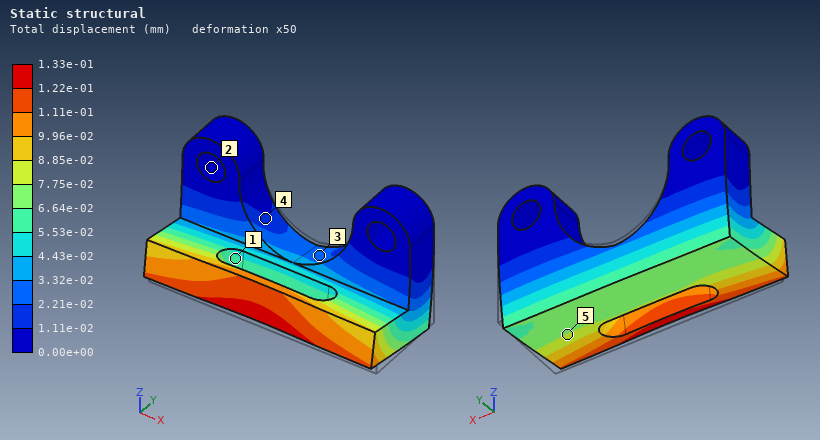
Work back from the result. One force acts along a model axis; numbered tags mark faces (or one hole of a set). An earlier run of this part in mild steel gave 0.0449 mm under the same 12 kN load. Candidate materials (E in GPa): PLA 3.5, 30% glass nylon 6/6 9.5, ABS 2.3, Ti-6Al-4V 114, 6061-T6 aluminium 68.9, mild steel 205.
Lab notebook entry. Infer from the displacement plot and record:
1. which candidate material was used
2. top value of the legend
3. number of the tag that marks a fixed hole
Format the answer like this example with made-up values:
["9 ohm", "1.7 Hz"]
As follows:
["6061-T6 aluminium", "1.33e-01 mm", "2"]
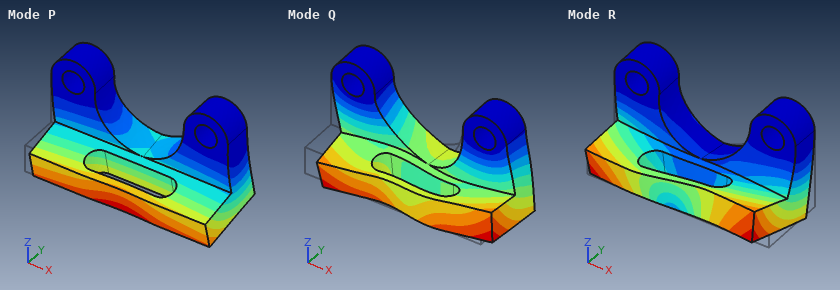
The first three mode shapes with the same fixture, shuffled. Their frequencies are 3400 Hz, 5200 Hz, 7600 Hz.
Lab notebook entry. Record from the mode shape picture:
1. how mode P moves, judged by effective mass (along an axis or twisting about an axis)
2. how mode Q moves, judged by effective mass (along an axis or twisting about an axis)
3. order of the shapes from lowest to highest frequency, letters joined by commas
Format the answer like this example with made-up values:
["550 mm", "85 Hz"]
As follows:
["along Y", "along X", "P, R, Q"]
